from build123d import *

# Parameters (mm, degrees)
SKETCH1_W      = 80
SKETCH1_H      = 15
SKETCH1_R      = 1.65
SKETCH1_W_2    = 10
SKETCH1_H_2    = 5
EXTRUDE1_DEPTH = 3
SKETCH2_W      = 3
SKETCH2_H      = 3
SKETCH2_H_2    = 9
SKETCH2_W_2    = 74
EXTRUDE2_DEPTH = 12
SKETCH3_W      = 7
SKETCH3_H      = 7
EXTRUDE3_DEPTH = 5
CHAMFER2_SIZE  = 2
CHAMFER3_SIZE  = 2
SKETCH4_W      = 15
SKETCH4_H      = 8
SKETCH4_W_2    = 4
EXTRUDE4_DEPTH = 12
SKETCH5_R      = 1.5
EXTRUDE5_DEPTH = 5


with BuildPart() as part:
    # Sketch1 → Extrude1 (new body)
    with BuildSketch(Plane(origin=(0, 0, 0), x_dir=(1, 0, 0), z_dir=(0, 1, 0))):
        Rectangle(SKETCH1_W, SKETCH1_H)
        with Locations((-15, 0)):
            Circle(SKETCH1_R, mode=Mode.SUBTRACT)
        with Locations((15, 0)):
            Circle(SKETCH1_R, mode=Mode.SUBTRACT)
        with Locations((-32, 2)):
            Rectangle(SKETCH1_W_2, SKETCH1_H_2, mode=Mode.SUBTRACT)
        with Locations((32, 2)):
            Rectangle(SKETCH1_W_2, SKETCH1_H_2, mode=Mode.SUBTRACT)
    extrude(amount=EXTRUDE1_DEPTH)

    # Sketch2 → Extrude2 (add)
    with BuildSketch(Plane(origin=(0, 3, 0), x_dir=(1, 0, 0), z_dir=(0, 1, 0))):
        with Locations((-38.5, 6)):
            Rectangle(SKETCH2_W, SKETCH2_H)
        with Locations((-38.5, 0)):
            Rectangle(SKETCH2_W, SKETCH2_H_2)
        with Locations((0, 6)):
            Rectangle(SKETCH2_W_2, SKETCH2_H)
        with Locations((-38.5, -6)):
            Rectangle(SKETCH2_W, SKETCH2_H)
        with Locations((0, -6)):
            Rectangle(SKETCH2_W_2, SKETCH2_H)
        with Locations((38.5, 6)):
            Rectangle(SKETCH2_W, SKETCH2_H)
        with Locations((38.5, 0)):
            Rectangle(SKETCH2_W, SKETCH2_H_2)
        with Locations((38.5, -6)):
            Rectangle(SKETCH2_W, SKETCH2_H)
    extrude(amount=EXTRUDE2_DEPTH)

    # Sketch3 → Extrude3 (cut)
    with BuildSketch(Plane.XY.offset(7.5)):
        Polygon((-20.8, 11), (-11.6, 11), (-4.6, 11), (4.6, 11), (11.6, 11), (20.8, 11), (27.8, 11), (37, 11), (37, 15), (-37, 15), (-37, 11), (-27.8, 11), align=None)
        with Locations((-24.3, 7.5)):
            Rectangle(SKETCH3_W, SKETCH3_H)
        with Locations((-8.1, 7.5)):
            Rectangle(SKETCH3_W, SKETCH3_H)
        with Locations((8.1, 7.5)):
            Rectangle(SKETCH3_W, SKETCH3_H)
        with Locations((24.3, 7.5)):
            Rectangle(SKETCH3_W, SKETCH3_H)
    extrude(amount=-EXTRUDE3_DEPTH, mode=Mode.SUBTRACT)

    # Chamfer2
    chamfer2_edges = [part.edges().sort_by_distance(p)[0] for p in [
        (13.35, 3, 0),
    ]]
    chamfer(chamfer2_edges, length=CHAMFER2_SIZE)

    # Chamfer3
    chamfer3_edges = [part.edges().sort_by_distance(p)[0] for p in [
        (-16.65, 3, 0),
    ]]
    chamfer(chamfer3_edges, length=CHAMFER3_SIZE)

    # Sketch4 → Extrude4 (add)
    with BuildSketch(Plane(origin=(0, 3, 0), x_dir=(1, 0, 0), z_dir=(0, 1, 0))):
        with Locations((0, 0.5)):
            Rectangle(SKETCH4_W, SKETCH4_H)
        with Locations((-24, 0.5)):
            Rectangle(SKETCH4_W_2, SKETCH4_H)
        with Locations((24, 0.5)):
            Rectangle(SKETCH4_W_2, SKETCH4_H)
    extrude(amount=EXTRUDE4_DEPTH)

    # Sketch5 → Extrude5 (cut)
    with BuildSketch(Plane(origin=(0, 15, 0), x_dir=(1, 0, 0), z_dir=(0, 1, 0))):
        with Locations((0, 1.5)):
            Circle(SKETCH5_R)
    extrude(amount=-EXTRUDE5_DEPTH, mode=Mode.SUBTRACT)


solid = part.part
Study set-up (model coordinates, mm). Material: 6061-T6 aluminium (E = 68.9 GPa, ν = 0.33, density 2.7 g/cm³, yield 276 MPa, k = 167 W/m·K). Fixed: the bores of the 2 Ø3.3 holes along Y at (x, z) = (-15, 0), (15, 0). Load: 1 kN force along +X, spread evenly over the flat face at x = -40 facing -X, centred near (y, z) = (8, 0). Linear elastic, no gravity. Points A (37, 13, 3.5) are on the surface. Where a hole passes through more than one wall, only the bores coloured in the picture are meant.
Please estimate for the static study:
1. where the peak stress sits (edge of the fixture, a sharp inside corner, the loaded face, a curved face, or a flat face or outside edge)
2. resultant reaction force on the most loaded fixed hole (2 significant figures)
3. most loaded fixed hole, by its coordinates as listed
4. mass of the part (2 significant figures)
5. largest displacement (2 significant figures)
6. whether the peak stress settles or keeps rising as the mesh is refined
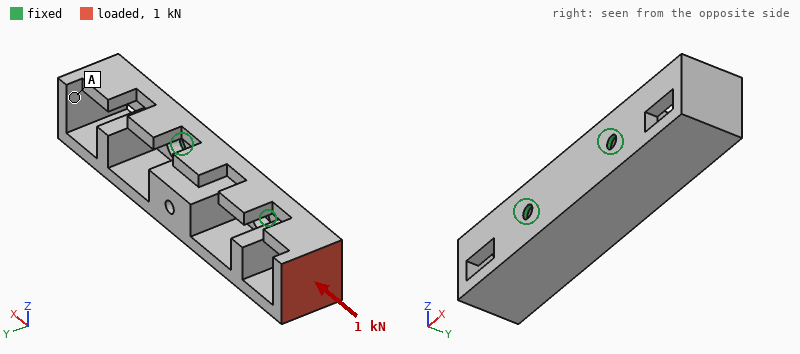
edge of the fixture
610 N
(-15, 0)
28 g
81 µm
keeps rising
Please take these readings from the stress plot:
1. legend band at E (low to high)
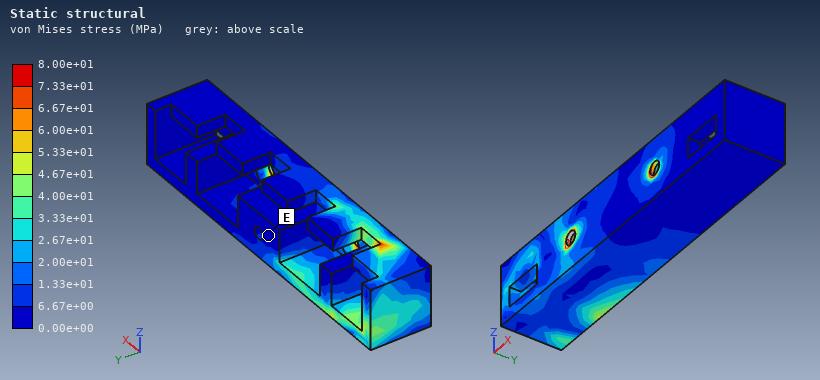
0.00e+00 to 6.67e+00 MPa
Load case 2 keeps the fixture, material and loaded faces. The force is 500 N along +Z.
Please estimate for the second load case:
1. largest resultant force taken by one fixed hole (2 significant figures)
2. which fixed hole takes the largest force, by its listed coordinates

850 N
(-15, 0)
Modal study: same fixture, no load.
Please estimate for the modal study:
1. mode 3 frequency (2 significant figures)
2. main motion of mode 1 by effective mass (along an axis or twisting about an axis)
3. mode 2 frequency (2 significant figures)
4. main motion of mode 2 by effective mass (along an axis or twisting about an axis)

5600 Hz
along Z
4700 Hz
twisting about Y
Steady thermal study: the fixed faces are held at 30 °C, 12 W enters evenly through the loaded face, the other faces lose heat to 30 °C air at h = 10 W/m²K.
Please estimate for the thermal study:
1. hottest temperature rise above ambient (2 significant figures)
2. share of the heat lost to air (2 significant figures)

29 K
3.8 %
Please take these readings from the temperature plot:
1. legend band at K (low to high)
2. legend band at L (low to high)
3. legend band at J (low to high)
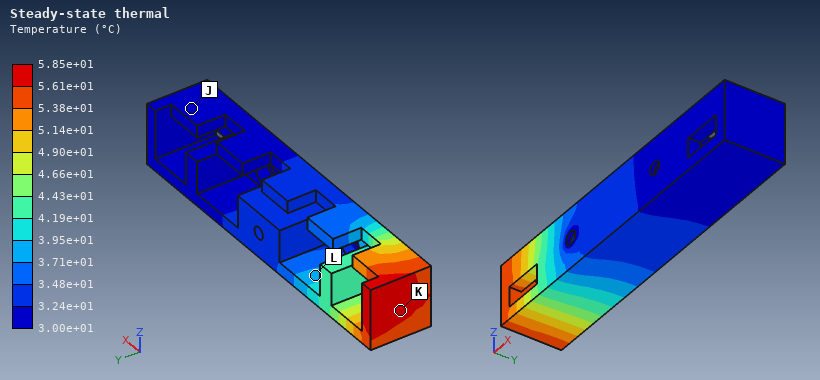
5.61e+01 to 5.85e+01 °C
3.71e+01 to 3.95e+01 °C
3.00e+01 to 3.24e+01 °C
